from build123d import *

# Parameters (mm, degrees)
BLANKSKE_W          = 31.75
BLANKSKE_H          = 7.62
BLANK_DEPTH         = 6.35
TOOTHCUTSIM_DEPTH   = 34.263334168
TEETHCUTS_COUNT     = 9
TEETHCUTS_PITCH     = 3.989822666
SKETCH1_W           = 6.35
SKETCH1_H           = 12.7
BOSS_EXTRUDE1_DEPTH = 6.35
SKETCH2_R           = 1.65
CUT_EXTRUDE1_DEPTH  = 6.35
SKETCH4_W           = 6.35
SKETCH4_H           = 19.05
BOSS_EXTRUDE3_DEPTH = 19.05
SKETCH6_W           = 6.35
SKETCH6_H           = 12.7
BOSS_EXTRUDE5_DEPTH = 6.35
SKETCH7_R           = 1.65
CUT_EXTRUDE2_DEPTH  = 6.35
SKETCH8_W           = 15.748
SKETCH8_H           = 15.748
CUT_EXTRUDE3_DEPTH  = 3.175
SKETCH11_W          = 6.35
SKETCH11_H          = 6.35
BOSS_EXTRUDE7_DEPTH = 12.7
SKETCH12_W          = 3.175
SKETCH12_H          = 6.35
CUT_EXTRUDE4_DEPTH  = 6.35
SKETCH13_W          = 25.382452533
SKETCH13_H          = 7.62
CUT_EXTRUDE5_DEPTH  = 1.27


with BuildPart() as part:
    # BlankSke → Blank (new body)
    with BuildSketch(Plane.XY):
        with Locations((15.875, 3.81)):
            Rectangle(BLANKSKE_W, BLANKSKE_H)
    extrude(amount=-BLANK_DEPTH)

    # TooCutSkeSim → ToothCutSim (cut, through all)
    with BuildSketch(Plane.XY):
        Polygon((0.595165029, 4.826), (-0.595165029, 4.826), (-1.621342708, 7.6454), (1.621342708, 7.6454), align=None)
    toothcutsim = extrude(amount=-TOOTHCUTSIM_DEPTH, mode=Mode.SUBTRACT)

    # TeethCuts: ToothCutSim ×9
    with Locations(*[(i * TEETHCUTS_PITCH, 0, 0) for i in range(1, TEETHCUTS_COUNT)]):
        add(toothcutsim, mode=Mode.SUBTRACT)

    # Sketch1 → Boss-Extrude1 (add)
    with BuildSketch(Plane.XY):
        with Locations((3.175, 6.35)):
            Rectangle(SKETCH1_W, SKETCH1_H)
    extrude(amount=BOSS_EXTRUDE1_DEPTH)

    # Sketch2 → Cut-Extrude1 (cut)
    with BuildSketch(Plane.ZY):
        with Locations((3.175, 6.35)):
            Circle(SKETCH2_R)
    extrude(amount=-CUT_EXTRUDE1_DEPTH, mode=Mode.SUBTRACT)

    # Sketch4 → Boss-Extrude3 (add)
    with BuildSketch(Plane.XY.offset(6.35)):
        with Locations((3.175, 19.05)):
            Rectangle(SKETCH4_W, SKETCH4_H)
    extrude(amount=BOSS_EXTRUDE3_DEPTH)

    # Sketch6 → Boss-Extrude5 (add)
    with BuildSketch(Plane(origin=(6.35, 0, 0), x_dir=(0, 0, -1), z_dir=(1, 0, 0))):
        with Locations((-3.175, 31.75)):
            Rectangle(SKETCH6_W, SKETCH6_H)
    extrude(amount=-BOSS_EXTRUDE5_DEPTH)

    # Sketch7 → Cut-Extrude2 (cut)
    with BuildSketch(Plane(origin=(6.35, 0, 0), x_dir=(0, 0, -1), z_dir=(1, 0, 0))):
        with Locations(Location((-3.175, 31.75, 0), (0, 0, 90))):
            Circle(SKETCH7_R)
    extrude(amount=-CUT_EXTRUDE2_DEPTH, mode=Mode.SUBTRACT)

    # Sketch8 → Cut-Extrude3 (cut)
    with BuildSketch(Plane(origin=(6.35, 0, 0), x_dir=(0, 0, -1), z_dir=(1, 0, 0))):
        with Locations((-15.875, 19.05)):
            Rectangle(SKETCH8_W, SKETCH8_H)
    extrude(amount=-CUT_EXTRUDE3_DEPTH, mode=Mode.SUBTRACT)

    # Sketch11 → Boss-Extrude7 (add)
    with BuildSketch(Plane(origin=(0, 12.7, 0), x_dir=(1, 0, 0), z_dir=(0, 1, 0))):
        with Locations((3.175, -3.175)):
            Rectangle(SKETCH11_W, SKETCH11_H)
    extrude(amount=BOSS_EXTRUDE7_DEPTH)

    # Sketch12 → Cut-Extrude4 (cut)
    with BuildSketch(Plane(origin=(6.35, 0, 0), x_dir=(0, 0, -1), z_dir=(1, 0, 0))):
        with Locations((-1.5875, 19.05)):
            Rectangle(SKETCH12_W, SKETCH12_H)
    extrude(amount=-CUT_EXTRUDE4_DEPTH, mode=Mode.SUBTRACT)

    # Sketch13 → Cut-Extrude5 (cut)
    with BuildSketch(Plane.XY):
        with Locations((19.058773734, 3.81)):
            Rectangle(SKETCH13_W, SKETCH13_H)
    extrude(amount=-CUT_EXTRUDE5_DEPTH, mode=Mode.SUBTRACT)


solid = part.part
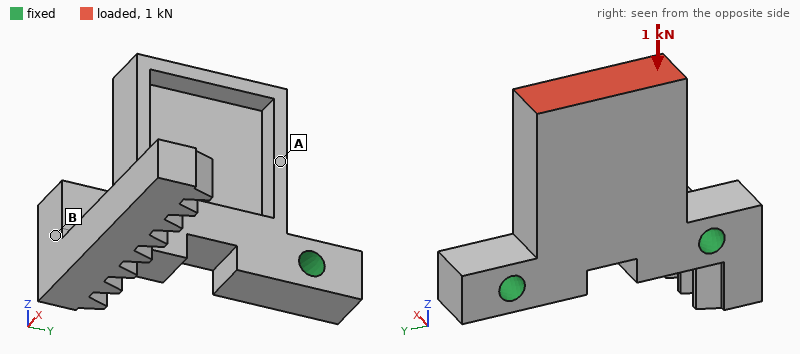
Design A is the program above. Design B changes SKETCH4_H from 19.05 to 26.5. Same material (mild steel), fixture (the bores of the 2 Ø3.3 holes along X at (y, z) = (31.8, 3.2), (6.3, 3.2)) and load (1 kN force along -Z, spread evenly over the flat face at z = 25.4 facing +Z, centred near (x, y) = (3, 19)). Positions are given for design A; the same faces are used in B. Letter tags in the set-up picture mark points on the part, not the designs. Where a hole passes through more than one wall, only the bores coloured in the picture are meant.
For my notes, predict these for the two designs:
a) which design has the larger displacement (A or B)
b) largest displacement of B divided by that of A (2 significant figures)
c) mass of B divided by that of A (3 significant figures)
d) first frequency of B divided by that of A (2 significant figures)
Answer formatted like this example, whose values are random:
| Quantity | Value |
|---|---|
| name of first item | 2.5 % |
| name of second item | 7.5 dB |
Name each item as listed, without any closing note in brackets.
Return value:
| Quantity | Value |
|---|---|
| which design has the larger displacement | A |
| largest displacement of B divided by that of A | 0.47 |
| mass of B divided by that of A | 1.23 |
| first frequency of B divided by that of A | 1.0 |
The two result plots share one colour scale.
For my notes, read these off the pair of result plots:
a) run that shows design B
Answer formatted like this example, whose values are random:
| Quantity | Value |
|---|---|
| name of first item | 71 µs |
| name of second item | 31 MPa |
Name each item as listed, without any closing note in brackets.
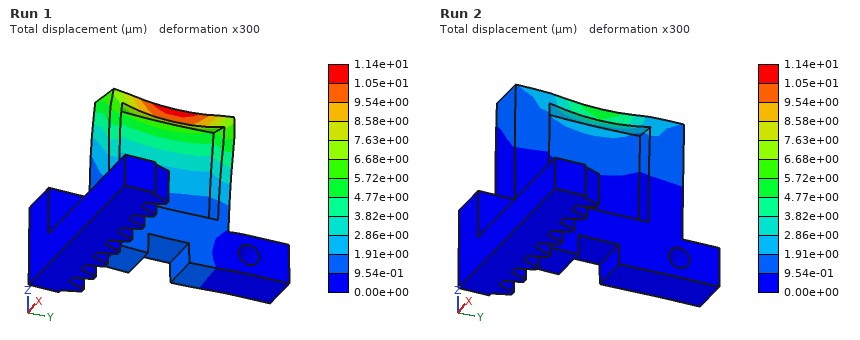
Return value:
| Quantity | Value |
|---|---|
| run that shows design B | Run 2 |
